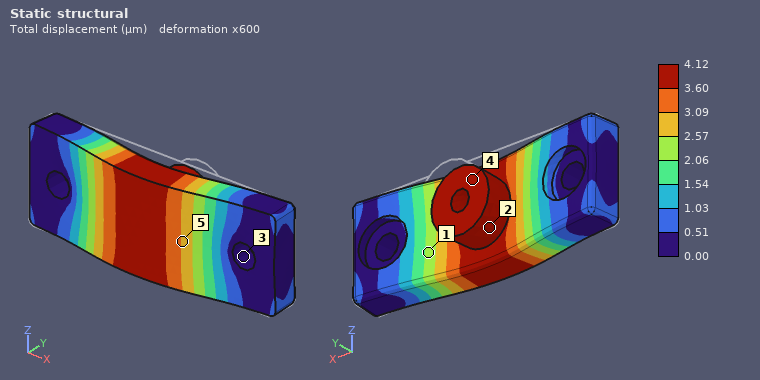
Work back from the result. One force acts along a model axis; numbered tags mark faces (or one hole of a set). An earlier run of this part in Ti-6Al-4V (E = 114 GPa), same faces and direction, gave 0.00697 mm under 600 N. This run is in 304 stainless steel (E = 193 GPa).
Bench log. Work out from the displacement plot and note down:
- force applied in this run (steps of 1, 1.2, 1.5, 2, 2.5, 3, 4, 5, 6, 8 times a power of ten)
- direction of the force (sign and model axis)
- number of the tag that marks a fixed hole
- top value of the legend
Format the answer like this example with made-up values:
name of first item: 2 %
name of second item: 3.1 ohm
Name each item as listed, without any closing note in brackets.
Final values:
force applied in this run: 600 N
direction of the force: -Y
number of the tag that marks a fixed hole: 3
top value of the legend: 4.12 µm
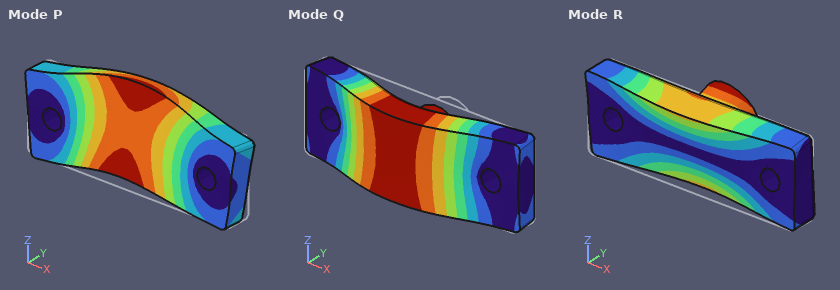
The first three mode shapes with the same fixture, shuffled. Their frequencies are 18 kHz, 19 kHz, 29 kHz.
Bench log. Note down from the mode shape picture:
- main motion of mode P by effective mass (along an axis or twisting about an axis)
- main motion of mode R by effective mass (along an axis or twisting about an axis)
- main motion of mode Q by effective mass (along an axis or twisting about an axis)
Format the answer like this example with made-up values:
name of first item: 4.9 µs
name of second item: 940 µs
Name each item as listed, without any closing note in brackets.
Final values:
main motion of mode P by effective mass: along Z
main motion of mode R by effective mass: along Z
main motion of mode Q by effective mass: along Y
